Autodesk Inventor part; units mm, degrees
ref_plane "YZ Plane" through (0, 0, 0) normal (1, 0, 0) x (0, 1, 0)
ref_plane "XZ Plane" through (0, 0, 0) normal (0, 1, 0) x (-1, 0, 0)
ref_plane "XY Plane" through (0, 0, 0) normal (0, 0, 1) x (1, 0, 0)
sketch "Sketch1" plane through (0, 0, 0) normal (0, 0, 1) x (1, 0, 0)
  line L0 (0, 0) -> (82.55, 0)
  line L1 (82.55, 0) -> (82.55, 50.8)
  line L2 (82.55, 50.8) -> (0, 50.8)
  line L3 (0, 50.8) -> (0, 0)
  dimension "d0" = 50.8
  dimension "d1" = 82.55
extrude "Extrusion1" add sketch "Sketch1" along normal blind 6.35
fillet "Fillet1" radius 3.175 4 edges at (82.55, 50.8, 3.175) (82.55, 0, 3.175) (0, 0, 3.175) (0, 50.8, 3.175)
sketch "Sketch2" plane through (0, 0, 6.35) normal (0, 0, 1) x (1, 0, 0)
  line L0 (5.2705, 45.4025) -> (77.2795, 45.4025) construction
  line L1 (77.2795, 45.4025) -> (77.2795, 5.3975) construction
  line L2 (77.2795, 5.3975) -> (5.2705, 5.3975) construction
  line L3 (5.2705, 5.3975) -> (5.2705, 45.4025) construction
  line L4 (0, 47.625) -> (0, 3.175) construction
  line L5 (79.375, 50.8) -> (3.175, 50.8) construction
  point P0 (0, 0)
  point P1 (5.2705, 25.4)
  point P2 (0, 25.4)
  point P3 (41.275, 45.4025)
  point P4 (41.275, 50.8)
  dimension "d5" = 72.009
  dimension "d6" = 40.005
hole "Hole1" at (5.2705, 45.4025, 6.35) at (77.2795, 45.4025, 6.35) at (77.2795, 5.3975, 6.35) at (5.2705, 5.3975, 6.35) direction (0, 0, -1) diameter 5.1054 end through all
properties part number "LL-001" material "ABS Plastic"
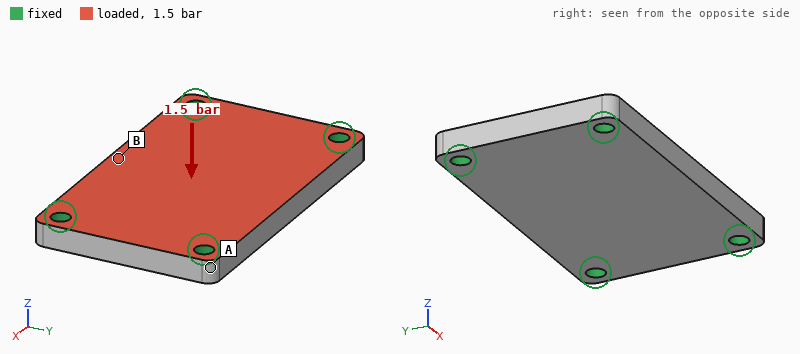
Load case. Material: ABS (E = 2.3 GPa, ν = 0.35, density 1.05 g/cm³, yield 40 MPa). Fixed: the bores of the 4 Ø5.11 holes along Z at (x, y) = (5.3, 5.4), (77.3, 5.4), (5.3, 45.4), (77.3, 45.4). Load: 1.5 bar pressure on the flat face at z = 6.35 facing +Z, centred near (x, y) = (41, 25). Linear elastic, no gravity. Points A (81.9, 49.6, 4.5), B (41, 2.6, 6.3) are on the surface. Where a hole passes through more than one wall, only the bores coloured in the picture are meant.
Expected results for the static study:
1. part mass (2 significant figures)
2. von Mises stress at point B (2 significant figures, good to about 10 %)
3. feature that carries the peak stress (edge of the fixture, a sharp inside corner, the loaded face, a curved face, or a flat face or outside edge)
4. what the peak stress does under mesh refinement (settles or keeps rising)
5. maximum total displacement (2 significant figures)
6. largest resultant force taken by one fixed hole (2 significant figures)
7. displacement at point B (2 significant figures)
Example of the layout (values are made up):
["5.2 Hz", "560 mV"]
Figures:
["27 g", "5.7 MPa", "edge of the fixture", "keeps rising", "0.28 mm", "150 N", "0.27 mm"]
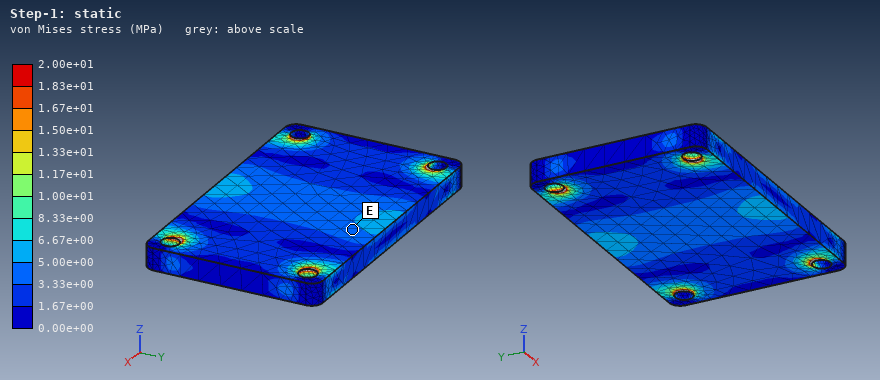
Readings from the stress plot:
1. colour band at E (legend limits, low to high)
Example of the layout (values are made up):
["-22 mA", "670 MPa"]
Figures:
["3.33e+00 to 5.00e+00 MPa"]
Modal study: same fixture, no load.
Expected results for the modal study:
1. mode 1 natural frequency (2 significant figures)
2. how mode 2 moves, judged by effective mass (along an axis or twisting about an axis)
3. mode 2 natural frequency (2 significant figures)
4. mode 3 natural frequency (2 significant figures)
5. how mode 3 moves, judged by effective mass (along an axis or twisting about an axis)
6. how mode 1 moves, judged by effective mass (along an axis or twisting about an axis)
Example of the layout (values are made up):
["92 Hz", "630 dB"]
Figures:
["1600 Hz", "twisting about X", "2500 Hz", "4100 Hz", "twisting about Y", "along Z"]
